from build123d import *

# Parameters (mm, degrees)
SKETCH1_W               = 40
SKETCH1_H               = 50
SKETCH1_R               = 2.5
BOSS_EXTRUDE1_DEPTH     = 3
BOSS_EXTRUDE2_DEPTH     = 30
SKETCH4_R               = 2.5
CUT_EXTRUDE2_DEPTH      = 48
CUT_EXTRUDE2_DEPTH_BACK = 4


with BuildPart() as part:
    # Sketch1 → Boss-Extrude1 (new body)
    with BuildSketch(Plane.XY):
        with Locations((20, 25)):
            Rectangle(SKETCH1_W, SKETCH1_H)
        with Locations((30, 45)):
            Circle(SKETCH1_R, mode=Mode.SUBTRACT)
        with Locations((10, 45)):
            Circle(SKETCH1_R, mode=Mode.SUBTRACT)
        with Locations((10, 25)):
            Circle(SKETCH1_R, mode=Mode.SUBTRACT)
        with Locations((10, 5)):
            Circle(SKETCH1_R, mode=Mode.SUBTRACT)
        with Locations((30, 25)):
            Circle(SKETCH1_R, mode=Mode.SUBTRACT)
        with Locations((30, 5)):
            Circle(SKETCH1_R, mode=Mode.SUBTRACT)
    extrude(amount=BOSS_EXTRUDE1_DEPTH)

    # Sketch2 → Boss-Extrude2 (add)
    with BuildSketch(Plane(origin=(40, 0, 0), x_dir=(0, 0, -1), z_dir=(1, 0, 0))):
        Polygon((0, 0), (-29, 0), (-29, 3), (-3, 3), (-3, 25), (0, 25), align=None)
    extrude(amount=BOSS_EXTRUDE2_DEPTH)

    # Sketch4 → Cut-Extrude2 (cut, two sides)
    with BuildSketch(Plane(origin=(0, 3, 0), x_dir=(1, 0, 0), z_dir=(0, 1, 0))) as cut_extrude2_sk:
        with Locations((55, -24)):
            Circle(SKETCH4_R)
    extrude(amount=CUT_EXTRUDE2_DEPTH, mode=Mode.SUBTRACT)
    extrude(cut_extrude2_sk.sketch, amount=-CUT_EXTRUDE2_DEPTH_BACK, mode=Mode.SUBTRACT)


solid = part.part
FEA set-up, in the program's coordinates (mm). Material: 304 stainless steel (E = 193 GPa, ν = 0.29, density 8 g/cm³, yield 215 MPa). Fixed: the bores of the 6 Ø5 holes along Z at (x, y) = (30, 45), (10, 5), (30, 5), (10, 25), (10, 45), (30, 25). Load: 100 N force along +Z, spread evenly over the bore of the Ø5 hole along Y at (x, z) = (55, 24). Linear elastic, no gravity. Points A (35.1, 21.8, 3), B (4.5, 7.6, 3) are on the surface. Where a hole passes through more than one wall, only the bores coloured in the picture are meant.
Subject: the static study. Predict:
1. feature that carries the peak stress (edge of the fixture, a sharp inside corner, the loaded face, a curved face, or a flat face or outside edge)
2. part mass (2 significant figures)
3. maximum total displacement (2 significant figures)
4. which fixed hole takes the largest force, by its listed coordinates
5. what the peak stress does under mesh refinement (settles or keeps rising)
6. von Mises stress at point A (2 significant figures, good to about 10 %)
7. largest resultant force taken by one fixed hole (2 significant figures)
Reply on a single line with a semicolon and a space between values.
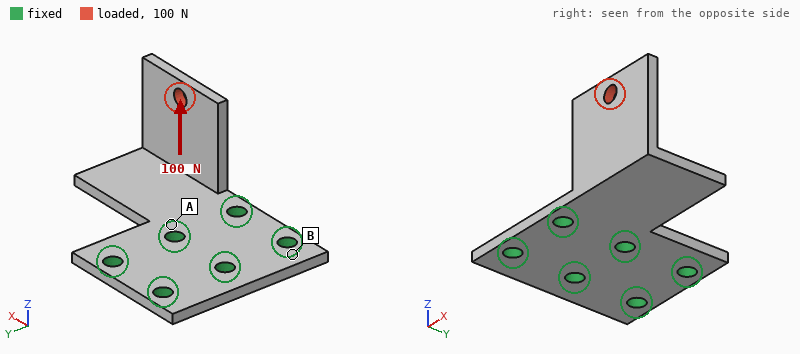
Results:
edge of the fixture; 81 g; 0.11 mm; (30, 5); keeps rising; 31 MPa; 120 N
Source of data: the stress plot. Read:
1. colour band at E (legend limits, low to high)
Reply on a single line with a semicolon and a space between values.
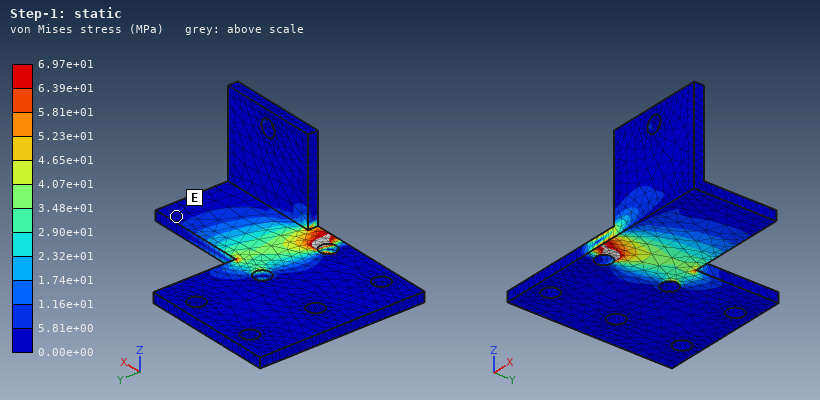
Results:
0.00e+00 to 5.81e+00 MPa
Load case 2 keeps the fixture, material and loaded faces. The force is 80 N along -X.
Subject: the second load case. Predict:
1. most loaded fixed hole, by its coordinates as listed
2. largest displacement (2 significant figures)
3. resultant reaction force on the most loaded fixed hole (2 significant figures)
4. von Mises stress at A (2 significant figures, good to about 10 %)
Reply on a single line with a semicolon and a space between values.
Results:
(30, 5); 0.11 mm; 86 N; 30 MPa
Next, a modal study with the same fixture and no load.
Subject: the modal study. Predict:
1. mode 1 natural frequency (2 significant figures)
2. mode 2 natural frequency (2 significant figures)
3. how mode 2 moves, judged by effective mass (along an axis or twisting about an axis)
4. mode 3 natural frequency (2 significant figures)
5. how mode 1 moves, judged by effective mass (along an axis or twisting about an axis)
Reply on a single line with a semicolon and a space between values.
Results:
1000 Hz; 1900 Hz; along Y; 5400 Hz; along Z
